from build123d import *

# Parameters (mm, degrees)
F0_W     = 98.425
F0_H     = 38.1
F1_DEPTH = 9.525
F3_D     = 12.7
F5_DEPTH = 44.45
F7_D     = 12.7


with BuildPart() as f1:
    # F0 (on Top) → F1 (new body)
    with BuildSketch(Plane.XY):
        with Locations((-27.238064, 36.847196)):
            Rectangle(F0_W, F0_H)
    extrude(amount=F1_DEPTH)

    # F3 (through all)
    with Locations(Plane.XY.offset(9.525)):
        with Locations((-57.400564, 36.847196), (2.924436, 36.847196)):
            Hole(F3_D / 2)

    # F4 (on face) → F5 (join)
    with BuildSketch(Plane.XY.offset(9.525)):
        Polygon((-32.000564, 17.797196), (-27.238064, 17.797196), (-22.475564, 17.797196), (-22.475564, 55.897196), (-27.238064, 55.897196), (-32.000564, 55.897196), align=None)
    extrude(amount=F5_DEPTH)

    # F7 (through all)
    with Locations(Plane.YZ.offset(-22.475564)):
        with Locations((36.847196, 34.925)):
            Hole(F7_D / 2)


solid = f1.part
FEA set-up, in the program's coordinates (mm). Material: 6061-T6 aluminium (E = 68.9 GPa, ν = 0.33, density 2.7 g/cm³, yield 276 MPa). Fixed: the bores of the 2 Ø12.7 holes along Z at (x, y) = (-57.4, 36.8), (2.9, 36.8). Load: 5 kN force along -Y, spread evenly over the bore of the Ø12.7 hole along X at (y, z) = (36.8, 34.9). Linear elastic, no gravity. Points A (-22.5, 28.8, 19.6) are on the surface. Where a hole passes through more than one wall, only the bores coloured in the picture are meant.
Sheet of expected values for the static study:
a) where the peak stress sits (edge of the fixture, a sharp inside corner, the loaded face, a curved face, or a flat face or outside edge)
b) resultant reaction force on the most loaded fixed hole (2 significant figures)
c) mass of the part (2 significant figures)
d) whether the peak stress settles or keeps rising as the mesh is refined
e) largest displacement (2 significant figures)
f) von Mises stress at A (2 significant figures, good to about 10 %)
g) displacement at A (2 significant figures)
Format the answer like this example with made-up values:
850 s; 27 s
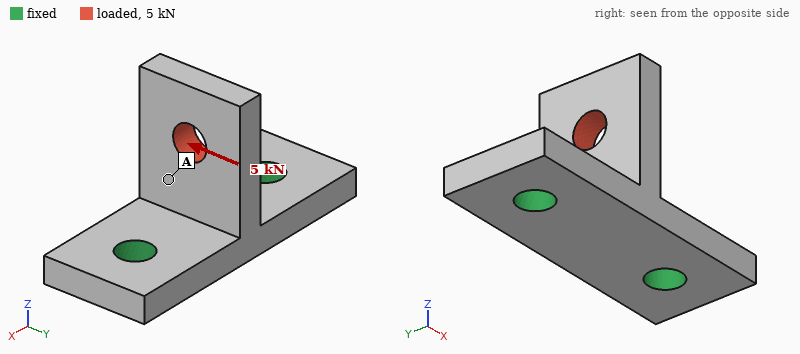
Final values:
edge of the fixture; 2.5 kN; 130 g; keeps rising; 0.32 mm; 30 MPa; 0.10 mm
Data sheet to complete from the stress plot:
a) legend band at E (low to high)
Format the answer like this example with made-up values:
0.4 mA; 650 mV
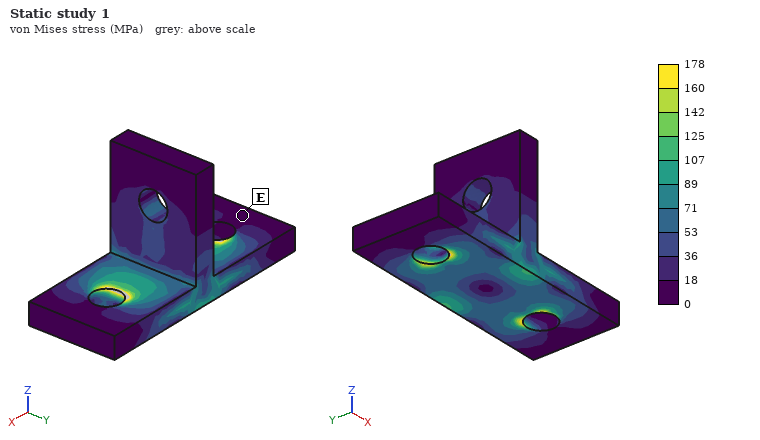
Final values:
0 to 18 MPa
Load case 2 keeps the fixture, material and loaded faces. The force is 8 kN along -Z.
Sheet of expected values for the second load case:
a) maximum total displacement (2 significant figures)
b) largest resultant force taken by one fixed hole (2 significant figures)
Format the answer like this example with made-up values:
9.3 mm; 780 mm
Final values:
56 µm; 4.0 kN
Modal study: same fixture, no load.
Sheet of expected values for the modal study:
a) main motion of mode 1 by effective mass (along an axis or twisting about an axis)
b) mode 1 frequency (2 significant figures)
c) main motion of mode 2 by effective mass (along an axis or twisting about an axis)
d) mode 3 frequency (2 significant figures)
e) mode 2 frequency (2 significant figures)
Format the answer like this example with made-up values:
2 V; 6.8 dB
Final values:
along X; 3200 Hz; along Y; 7900 Hz; 3800 Hz
